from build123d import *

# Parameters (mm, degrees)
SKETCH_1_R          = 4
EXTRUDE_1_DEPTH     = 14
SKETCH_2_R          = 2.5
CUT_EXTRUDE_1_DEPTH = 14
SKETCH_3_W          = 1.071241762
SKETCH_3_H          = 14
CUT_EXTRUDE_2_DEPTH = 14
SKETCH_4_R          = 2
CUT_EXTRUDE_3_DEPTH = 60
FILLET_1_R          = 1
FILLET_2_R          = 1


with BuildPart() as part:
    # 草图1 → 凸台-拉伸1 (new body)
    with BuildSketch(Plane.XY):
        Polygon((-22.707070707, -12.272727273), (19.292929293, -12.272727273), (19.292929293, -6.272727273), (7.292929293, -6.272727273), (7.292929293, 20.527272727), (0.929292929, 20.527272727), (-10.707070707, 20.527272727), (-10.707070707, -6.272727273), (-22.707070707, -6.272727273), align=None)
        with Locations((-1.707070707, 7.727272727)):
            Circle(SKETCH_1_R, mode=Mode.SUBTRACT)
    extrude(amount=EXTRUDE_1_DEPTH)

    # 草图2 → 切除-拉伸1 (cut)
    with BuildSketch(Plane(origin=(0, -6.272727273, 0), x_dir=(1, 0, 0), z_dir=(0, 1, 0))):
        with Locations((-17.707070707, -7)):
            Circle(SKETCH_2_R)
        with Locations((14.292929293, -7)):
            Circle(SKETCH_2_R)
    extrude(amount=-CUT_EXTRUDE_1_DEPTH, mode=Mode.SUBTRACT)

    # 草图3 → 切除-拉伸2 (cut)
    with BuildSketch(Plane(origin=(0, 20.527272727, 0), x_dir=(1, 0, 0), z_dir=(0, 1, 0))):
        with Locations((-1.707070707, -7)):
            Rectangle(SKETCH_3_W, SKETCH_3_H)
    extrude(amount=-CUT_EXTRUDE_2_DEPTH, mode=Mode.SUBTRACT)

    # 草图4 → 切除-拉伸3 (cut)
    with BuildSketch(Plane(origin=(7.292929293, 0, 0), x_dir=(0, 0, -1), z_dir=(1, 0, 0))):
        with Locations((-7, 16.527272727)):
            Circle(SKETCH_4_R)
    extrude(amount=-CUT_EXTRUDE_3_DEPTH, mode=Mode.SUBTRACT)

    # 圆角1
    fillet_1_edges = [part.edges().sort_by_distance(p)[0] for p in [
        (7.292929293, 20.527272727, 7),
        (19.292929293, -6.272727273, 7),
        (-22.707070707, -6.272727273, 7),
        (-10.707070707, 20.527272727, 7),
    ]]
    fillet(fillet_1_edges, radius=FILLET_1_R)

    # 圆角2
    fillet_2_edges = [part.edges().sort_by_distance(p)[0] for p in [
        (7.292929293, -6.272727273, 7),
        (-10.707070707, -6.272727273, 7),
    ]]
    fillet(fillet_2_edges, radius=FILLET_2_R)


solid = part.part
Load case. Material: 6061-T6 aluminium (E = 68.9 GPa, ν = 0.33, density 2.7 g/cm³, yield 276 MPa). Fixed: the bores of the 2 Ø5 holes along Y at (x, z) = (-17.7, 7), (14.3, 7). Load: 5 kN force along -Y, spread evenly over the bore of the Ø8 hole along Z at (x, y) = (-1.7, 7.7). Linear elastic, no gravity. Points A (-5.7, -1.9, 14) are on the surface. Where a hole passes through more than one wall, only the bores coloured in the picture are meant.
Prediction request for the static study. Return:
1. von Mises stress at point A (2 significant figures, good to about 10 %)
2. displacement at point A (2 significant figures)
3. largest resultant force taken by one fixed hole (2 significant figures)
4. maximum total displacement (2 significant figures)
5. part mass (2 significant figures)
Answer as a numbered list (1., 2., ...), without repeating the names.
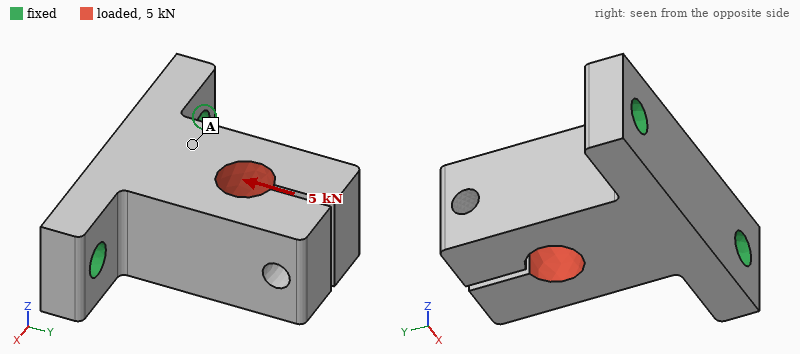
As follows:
1. 35 MPa
2. 20 µm
3. 2.7 kN
4. 66 µm
5. 24 g
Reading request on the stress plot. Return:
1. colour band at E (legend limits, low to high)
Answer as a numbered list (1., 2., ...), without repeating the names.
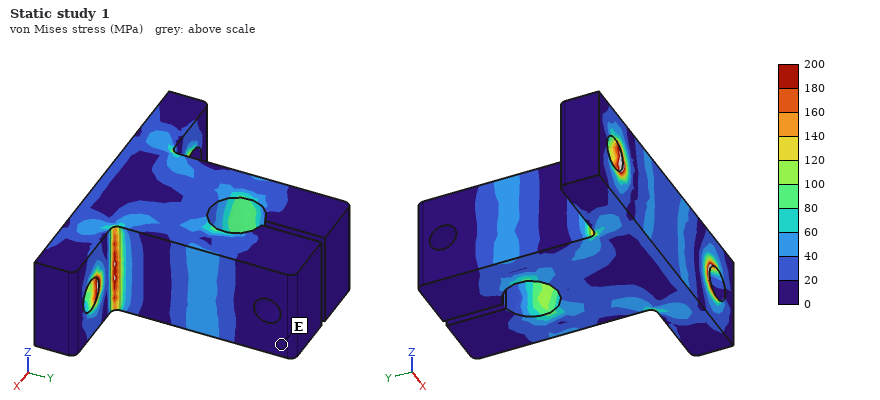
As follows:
1. 0 to 20 MPa
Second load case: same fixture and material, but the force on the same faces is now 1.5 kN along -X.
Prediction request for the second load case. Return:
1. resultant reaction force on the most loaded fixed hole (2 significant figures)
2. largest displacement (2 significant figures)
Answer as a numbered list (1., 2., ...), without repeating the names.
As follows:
1. 1.3 kN
2. 44 µm
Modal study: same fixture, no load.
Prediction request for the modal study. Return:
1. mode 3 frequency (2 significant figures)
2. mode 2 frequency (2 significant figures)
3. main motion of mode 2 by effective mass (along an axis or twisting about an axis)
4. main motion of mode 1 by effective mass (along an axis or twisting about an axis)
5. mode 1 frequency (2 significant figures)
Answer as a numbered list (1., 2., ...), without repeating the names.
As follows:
1. 10 kHz
2. 8300 Hz
3. along X
4. along Z
5. 5000 Hz
